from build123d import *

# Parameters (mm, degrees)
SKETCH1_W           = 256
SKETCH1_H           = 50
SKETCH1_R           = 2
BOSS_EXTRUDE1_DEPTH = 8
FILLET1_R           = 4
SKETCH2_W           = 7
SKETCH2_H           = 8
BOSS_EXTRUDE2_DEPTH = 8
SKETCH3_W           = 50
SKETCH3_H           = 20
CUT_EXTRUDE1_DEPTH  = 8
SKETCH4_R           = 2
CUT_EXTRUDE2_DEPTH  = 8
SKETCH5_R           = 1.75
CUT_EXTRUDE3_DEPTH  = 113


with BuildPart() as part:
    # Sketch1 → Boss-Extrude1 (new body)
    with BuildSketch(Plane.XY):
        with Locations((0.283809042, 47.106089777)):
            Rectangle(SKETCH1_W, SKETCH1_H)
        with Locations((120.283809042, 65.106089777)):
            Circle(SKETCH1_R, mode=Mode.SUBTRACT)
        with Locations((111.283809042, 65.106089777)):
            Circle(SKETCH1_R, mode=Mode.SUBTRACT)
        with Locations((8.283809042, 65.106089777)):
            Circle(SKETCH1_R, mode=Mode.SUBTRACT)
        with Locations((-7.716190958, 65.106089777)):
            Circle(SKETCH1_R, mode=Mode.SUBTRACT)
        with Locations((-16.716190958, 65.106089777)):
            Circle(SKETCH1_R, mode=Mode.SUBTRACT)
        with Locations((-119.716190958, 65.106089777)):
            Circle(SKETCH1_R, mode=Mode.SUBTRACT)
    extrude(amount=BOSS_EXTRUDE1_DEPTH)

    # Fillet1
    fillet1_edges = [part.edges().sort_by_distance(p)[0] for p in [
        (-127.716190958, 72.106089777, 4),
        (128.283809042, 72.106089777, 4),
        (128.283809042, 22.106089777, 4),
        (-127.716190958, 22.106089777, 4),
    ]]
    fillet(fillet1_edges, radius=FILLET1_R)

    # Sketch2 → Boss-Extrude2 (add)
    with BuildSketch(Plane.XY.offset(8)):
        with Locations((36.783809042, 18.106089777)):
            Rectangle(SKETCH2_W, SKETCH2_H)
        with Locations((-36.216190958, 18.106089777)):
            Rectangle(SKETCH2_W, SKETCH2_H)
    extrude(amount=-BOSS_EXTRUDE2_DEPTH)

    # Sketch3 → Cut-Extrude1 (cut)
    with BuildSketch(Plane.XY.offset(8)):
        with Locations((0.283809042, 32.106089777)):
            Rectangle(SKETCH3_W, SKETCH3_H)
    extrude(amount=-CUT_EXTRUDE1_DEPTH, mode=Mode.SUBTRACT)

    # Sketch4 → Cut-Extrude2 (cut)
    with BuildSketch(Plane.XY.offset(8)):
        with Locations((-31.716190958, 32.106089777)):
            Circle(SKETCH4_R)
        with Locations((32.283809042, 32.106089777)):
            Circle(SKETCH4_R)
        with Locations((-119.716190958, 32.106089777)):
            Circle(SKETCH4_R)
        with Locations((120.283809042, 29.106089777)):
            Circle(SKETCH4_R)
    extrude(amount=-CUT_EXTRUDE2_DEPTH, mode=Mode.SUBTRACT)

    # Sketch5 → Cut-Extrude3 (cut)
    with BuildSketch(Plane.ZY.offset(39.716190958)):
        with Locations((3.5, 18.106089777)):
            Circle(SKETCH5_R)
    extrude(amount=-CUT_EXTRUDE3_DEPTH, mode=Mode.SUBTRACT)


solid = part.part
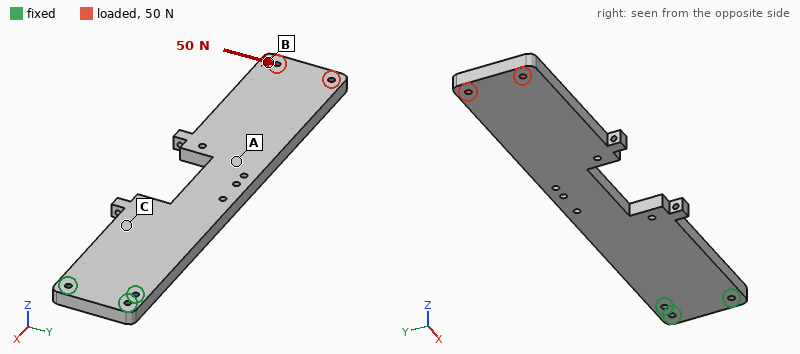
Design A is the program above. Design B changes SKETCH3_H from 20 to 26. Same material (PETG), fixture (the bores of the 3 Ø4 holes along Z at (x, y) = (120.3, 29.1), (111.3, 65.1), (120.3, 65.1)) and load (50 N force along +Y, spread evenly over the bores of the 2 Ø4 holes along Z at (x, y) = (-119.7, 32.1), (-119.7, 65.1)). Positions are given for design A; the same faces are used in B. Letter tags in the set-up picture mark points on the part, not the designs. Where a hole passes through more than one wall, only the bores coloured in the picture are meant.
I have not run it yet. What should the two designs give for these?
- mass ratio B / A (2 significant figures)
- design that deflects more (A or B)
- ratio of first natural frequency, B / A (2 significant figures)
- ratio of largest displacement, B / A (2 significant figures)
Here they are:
0.99
B
0.98
1.2
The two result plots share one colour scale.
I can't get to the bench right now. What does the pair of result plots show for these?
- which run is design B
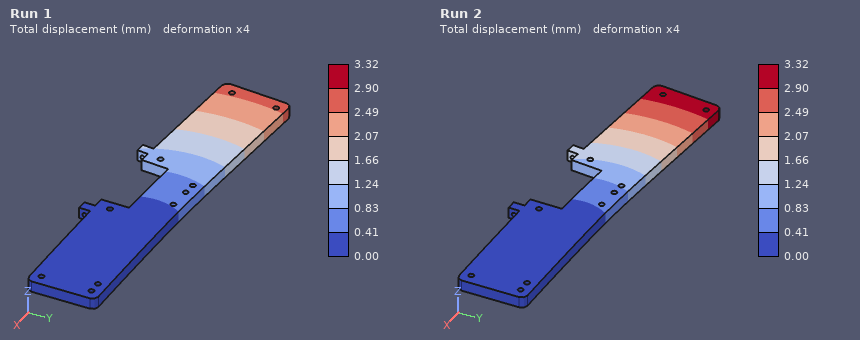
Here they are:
Run 2
